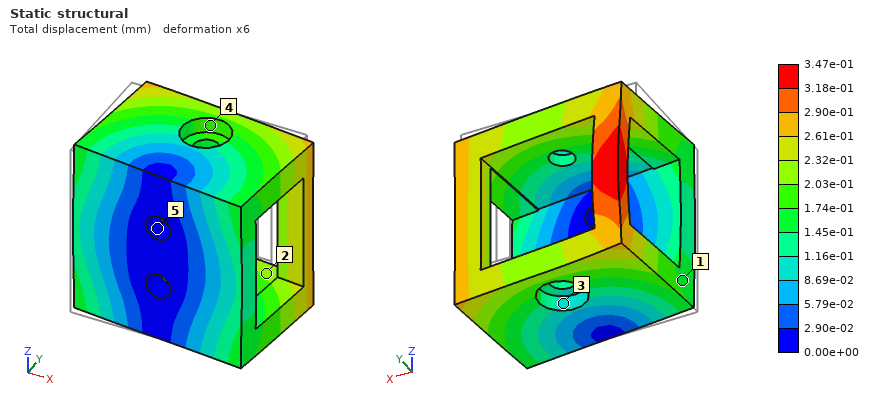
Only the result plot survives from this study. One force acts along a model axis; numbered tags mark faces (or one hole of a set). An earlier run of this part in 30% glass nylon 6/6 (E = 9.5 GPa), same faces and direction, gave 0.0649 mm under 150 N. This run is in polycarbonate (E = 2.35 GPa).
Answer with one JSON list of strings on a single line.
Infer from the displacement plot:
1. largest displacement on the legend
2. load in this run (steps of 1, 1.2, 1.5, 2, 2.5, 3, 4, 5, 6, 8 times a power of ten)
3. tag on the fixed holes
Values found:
["3.47e-01 mm", "200 N", "5"]
